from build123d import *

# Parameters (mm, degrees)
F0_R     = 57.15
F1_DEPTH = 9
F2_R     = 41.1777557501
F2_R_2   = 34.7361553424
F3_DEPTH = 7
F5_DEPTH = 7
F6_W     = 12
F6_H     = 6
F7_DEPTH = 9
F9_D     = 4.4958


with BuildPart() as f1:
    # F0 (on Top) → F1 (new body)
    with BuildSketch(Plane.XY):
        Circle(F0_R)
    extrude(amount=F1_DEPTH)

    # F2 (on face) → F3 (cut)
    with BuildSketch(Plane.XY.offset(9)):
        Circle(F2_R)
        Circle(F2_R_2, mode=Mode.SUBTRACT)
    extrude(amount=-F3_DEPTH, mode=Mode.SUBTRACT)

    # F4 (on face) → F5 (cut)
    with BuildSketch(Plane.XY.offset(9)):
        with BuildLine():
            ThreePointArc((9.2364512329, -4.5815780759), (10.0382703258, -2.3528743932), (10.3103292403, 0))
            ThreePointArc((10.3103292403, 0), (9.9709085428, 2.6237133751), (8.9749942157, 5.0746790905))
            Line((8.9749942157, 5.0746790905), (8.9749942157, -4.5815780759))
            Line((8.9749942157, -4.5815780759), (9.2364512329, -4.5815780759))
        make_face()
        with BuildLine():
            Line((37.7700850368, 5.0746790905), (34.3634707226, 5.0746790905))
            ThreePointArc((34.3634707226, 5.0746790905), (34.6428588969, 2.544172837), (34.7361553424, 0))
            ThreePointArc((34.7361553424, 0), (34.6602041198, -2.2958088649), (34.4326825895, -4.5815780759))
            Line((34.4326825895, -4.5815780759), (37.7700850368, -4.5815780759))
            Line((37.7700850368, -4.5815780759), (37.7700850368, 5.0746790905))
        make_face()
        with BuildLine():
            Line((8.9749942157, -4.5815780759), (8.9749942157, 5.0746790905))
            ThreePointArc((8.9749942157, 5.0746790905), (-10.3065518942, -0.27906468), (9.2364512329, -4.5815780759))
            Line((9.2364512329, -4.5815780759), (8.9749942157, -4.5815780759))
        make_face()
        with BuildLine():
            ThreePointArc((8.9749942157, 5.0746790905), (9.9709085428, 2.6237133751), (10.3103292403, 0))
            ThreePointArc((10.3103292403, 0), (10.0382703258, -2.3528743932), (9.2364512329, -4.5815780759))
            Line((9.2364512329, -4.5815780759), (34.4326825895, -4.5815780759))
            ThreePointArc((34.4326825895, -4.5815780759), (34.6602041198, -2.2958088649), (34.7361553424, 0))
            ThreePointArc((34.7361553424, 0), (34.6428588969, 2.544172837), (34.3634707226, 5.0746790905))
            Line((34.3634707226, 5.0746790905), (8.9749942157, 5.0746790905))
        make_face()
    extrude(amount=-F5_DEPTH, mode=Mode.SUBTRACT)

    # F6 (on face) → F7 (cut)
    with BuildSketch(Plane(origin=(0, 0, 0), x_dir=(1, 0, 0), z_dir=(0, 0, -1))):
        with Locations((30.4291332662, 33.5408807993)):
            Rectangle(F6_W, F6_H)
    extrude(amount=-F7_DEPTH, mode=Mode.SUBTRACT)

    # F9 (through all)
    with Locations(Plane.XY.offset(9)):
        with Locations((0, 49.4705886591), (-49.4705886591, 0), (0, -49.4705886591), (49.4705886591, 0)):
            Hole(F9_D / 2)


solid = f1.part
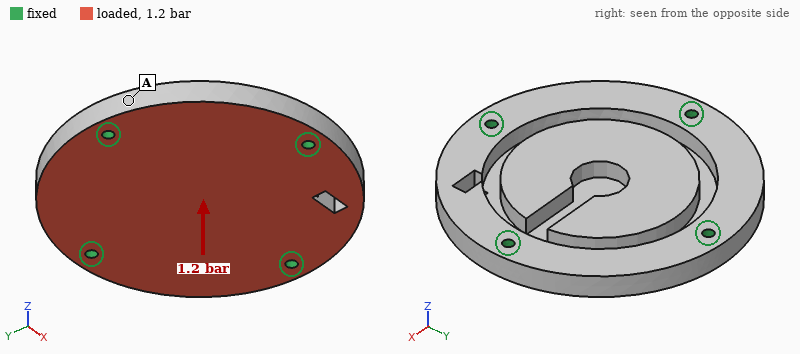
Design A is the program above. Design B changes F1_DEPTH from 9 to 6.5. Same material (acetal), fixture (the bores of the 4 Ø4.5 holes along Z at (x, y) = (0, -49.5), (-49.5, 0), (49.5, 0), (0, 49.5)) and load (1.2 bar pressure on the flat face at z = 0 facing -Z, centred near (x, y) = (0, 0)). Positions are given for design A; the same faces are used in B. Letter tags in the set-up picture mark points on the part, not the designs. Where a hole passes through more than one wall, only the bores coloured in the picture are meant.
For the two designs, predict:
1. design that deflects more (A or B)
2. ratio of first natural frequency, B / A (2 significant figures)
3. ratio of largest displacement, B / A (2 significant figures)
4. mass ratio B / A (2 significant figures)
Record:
B
0.84
1.9
0.74
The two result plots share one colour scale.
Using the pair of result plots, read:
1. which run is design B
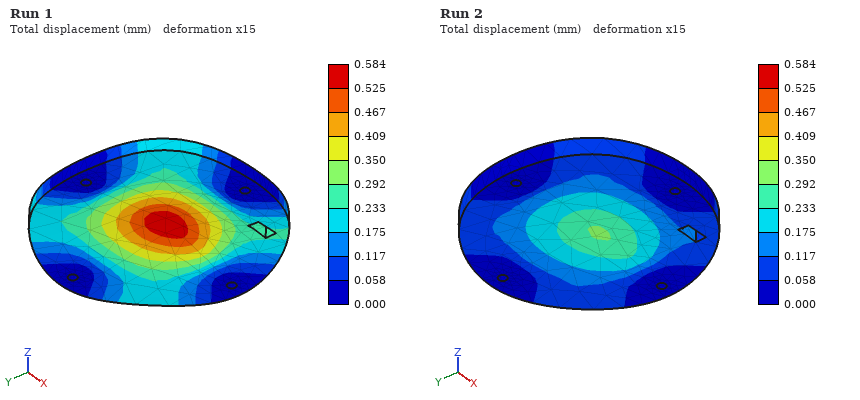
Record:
Run 1
